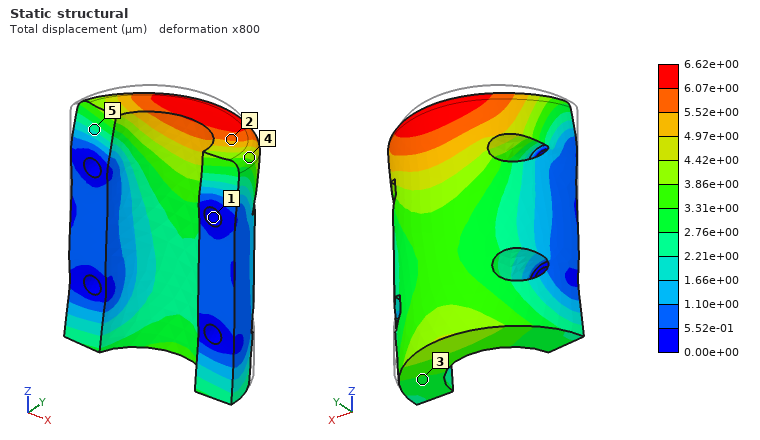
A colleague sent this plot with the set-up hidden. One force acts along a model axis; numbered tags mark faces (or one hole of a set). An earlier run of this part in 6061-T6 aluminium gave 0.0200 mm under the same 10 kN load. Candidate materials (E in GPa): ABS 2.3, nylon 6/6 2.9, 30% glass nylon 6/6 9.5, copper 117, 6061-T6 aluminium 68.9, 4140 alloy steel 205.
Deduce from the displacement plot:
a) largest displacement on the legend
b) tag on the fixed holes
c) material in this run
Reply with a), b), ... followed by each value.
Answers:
a) 6.62e+00 µm
b) 1
c) 4140 alloy steel
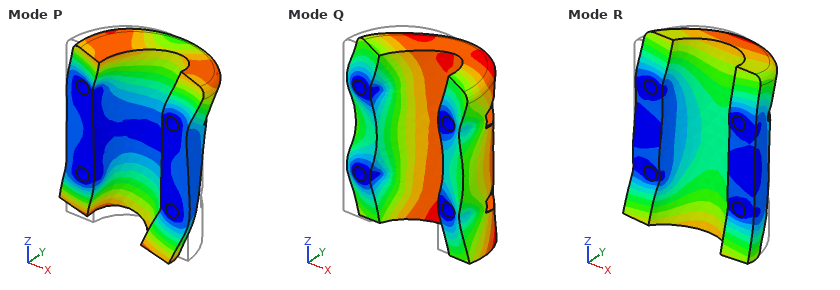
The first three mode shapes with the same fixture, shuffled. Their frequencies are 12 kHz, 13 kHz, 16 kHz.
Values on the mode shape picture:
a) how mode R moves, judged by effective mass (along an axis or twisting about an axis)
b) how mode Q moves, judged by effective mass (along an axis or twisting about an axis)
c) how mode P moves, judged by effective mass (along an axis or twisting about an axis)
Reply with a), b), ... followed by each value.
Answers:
a) along Z
b) along X
c) twisting about Y
